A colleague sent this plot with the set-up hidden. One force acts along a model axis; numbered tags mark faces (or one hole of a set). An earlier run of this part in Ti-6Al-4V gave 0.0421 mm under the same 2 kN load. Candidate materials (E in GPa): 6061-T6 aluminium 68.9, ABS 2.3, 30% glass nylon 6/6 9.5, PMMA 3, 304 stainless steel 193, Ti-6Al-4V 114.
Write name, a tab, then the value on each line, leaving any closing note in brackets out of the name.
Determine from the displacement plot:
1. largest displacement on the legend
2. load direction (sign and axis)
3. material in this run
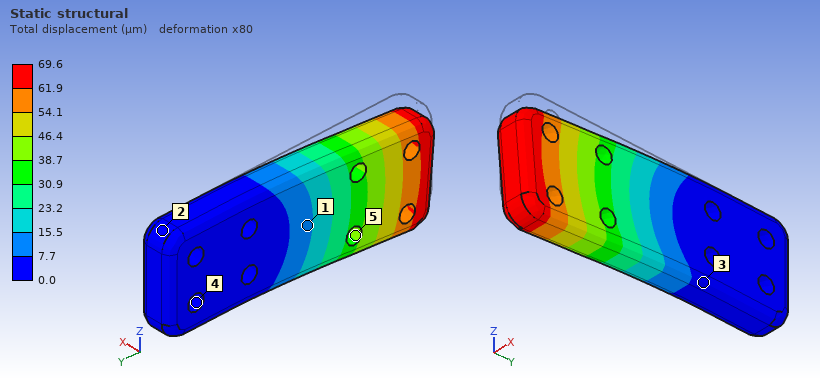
largest displacement on the legend	69.6 µm
load direction	-Z
material in this run	6061-T6 aluminium
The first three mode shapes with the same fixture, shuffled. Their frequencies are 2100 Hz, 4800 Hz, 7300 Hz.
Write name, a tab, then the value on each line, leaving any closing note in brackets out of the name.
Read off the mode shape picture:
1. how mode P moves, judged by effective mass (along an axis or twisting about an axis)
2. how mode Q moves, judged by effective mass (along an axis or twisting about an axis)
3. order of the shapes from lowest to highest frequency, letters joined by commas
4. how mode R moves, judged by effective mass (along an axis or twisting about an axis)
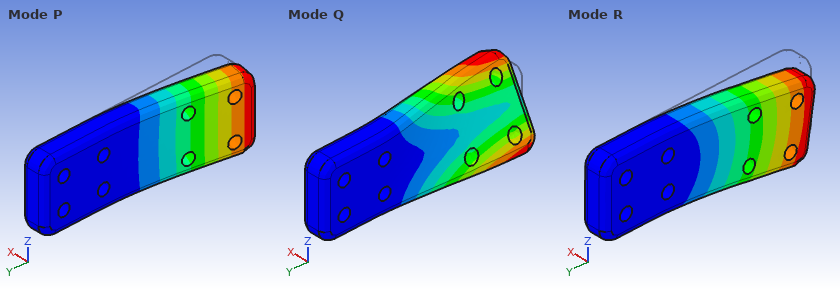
how mode P moves, judged by effective mass	along X
how mode Q moves, judged by effective mass	twisting about Y
order of the shapes from lowest to highest frequency, letters joined by commas	P, R, Q
how mode R moves, judged by effective mass	along Z
